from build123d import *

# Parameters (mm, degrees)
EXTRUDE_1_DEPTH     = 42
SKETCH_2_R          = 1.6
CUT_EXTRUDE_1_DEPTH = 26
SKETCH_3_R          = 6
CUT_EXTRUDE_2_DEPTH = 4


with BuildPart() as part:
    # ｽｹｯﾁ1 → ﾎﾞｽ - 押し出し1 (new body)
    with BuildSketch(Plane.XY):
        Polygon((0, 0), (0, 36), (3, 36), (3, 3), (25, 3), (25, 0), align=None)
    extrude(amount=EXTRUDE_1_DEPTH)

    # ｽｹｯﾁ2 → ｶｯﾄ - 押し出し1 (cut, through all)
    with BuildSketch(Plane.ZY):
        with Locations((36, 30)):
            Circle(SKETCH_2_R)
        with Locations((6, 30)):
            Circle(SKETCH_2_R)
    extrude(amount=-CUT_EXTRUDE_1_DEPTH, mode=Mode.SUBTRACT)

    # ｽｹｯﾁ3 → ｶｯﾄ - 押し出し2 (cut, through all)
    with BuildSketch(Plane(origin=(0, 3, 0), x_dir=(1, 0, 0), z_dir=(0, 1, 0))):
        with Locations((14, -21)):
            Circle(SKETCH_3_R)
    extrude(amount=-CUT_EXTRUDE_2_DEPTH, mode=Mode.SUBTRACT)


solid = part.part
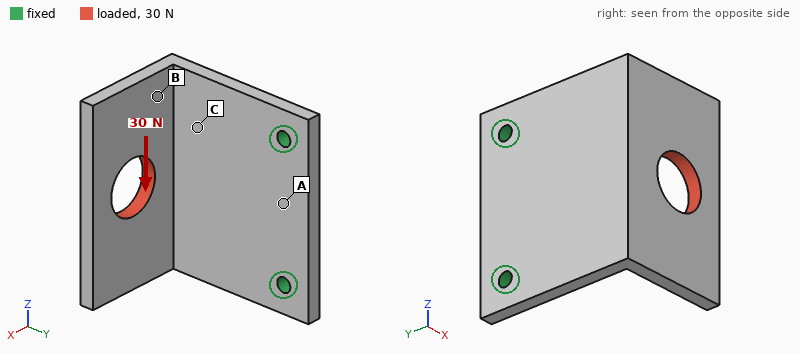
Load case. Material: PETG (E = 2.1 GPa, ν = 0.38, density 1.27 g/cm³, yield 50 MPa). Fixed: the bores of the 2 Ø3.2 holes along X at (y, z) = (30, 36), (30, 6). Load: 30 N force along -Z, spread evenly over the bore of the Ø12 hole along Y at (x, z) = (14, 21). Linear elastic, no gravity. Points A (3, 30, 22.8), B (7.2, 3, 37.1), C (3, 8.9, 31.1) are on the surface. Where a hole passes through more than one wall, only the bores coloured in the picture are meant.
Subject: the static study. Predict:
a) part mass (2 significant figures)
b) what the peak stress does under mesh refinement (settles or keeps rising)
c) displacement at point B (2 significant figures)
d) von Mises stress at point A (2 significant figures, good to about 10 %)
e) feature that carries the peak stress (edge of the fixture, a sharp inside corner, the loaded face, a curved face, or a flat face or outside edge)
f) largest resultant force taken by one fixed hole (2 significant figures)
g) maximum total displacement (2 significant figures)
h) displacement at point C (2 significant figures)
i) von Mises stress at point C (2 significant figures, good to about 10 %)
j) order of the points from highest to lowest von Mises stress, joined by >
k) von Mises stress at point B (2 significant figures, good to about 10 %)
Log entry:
8.8 g
keeps rising
0.32 mm
0.95 MPa
edge of the fixture
33 N
0.63 mm
0.14 mm
3.8 MPa
C > B > A
2.4 MPa
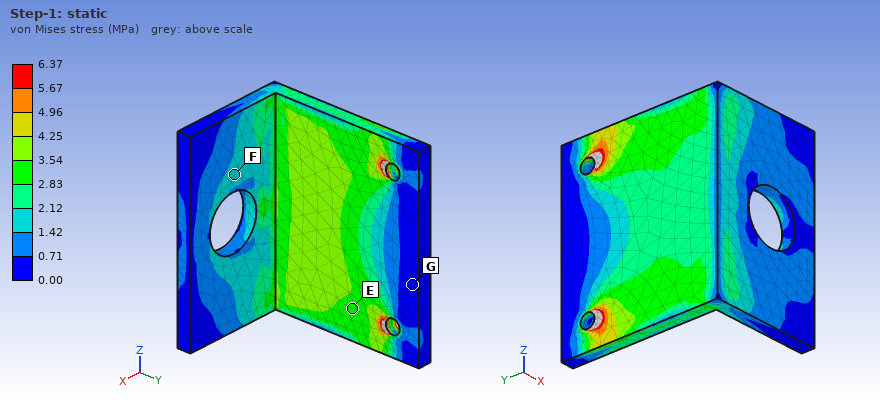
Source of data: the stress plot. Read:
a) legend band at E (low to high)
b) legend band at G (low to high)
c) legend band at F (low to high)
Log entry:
2.83 to 3.54 MPa
0.00 to 0.71 MPa
1.42 to 2.12 MPa
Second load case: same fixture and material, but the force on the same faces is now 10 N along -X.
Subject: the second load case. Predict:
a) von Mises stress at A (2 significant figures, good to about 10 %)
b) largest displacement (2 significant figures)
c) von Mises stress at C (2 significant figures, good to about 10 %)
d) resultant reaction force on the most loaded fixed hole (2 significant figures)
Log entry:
1.3 MPa
0.68 mm
1.1 MPa
5.0 N
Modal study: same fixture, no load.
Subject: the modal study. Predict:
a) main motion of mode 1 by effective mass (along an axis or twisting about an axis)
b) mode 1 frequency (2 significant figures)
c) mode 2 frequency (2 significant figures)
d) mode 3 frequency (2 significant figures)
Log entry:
along X
310 Hz
590 Hz
920 Hz
